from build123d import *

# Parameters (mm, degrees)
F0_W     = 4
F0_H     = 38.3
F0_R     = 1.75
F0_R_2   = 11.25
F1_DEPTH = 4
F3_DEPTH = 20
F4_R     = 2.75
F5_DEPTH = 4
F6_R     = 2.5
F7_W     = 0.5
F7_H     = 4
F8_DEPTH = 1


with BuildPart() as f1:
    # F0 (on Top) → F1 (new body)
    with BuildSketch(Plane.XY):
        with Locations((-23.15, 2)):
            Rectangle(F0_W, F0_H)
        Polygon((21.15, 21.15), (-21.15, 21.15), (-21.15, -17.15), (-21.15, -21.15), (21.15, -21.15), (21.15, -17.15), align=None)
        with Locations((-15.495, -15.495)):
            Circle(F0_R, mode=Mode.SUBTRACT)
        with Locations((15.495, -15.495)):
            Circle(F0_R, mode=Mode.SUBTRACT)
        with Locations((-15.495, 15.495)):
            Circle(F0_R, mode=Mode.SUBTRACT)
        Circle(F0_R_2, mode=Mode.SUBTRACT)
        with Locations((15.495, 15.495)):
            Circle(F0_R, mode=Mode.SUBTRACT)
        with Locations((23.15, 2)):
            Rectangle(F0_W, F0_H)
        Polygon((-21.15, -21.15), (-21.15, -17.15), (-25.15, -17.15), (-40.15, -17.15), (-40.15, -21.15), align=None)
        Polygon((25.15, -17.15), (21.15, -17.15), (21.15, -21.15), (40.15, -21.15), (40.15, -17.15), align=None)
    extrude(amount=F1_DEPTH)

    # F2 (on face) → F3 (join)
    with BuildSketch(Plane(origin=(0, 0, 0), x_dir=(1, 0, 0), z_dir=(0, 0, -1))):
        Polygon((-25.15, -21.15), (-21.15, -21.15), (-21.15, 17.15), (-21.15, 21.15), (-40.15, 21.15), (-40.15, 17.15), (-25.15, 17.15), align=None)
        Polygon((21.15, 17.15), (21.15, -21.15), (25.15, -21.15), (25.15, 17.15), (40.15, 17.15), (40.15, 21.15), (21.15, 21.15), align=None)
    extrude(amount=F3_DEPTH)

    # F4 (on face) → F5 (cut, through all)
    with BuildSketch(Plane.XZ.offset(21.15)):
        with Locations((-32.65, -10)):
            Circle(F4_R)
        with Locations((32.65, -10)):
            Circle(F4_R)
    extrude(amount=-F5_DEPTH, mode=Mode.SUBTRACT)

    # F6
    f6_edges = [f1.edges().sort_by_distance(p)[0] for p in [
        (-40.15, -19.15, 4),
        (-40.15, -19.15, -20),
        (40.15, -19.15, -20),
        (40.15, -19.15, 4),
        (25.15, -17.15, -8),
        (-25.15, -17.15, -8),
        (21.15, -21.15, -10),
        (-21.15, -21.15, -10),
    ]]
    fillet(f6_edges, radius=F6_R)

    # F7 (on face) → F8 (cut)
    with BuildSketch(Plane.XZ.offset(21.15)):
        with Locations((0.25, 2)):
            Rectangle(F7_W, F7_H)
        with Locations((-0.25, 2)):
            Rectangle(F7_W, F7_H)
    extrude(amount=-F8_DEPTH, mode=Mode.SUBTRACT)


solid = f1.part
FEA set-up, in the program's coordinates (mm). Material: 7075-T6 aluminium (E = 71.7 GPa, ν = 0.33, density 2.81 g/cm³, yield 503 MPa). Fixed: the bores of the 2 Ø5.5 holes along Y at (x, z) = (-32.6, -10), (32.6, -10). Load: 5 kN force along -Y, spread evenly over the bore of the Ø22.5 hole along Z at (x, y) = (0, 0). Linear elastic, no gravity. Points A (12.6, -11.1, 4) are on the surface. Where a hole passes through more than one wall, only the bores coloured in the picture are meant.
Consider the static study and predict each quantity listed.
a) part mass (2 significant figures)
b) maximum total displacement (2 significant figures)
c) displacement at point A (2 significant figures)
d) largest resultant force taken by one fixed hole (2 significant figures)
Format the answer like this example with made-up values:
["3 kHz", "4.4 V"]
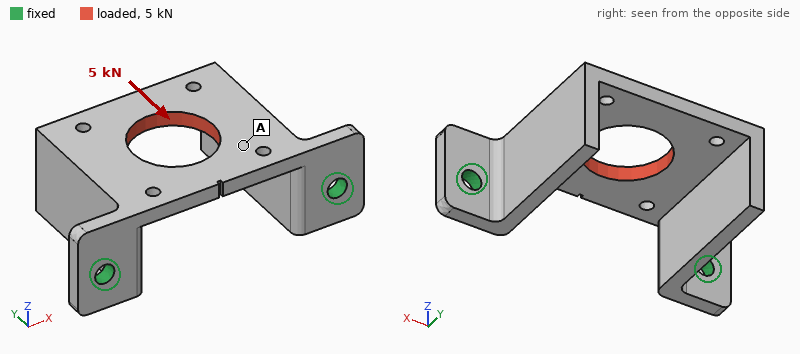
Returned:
["46 g", "0.57 mm", "0.25 mm", "2.7 kN"]
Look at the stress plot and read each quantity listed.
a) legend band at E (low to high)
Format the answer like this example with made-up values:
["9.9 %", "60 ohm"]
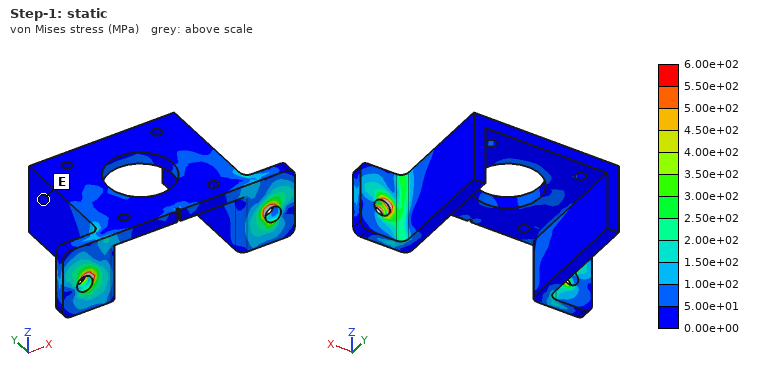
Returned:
["0.00e+00 to 5.00e+01 MPa"]
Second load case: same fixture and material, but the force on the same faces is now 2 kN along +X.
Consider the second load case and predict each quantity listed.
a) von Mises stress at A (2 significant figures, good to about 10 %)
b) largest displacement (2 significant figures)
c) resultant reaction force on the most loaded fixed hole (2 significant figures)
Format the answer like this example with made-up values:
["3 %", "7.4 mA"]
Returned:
["13 MPa", "0.11 mm", "1.2 kN"]
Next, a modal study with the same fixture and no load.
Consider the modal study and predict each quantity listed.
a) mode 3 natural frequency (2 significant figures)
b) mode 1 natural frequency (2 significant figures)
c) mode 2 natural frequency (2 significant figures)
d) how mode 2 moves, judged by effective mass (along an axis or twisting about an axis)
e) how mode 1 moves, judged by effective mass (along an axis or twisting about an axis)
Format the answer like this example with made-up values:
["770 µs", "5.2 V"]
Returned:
["4700 Hz", "2100 Hz", "2800 Hz", "along X", "along Z"]
